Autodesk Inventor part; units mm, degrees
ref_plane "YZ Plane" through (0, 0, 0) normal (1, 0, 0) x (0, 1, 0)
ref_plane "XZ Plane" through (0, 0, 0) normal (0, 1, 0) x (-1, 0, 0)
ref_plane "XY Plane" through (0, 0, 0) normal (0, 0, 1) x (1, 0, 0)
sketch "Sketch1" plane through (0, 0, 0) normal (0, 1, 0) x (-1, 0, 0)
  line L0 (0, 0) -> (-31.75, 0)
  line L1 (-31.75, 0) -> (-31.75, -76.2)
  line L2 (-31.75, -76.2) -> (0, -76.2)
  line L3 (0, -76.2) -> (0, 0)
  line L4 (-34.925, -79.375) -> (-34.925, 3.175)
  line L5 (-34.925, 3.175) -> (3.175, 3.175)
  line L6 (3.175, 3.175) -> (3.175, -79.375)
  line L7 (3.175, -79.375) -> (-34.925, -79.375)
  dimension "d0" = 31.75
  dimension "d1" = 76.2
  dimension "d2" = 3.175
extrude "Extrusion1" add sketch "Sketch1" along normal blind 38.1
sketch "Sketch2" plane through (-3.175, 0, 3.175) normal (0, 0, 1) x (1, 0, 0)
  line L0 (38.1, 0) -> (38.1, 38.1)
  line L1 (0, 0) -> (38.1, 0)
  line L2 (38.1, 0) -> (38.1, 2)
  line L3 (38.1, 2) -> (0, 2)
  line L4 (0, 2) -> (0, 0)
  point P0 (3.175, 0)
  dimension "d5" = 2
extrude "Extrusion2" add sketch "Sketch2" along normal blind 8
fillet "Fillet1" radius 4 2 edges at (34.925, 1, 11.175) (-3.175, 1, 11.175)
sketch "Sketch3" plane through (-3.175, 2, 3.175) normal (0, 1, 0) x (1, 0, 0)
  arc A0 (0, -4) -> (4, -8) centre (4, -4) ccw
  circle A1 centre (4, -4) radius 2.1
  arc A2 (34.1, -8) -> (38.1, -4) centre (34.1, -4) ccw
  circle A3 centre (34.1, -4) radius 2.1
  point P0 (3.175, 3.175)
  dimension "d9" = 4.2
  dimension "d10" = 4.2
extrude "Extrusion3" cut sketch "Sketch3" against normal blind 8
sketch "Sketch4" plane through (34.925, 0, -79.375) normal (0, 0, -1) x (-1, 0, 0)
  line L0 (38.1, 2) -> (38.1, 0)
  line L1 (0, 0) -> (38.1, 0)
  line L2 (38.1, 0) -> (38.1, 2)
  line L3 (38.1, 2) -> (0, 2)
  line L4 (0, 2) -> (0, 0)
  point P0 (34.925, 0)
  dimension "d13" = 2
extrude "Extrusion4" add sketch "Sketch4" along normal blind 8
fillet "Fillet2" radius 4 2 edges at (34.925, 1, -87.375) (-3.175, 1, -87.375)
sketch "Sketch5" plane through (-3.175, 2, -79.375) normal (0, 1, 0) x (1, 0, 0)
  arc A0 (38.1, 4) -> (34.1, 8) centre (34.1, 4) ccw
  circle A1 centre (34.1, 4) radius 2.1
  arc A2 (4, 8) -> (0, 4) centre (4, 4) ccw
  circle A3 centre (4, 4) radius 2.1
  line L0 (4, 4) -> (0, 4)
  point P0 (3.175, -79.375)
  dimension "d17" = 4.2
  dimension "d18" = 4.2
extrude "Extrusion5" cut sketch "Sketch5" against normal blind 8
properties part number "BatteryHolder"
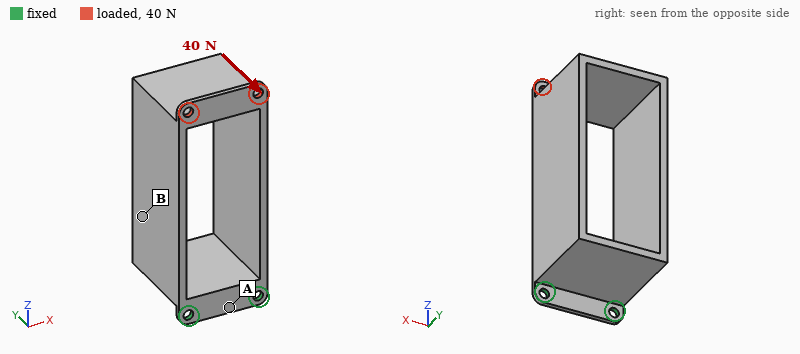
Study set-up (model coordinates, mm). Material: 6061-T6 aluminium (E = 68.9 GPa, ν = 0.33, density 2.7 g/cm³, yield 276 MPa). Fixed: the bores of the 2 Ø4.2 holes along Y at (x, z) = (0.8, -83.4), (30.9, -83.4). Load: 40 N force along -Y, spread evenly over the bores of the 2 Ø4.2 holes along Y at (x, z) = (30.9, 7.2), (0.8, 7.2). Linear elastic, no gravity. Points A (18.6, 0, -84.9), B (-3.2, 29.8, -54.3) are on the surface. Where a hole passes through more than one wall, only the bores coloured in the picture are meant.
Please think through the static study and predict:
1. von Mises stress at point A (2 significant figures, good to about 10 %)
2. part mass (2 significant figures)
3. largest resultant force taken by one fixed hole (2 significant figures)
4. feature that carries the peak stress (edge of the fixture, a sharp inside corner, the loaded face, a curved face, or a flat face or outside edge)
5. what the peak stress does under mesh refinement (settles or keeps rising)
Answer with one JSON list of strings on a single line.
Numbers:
["36 MPa", "78 g", "44 N", "edge of the fixture", "keeps rising"]
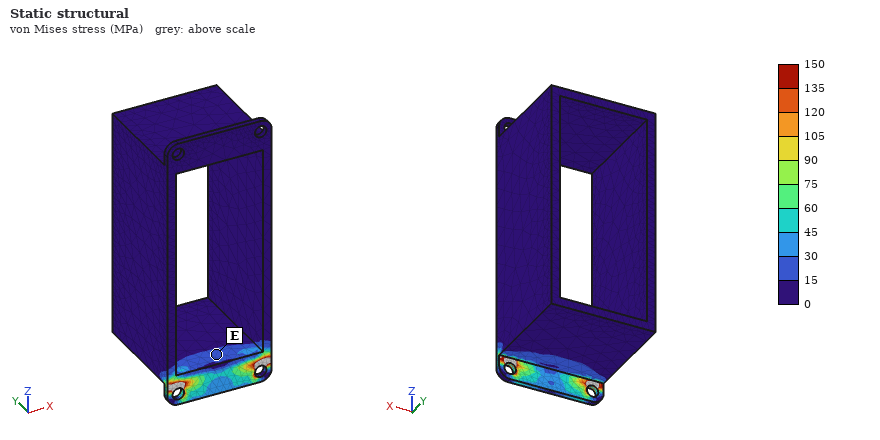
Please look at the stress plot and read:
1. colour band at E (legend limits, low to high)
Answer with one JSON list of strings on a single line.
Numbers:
["15 to 30 MPa"]
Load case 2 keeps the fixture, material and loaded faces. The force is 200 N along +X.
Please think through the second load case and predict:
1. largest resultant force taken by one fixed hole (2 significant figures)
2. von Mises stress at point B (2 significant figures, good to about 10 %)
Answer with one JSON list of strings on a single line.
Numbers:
["530 N", "32 MPa"]
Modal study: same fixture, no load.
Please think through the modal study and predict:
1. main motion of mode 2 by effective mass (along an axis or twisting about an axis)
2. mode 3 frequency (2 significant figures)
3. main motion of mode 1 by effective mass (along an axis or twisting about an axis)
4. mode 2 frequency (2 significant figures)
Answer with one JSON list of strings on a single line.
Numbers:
["along X", "1100 Hz", "along Y", "420 Hz"]
